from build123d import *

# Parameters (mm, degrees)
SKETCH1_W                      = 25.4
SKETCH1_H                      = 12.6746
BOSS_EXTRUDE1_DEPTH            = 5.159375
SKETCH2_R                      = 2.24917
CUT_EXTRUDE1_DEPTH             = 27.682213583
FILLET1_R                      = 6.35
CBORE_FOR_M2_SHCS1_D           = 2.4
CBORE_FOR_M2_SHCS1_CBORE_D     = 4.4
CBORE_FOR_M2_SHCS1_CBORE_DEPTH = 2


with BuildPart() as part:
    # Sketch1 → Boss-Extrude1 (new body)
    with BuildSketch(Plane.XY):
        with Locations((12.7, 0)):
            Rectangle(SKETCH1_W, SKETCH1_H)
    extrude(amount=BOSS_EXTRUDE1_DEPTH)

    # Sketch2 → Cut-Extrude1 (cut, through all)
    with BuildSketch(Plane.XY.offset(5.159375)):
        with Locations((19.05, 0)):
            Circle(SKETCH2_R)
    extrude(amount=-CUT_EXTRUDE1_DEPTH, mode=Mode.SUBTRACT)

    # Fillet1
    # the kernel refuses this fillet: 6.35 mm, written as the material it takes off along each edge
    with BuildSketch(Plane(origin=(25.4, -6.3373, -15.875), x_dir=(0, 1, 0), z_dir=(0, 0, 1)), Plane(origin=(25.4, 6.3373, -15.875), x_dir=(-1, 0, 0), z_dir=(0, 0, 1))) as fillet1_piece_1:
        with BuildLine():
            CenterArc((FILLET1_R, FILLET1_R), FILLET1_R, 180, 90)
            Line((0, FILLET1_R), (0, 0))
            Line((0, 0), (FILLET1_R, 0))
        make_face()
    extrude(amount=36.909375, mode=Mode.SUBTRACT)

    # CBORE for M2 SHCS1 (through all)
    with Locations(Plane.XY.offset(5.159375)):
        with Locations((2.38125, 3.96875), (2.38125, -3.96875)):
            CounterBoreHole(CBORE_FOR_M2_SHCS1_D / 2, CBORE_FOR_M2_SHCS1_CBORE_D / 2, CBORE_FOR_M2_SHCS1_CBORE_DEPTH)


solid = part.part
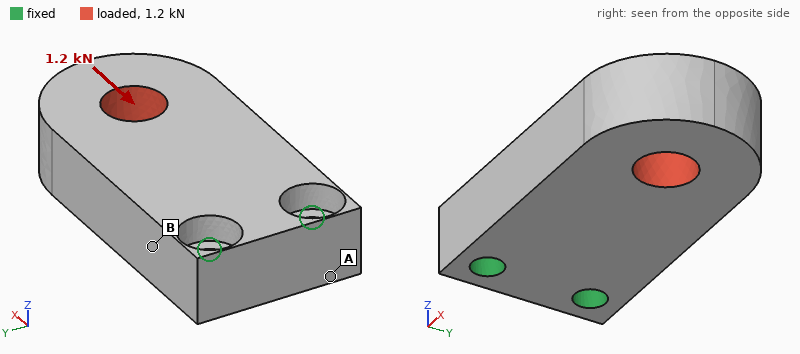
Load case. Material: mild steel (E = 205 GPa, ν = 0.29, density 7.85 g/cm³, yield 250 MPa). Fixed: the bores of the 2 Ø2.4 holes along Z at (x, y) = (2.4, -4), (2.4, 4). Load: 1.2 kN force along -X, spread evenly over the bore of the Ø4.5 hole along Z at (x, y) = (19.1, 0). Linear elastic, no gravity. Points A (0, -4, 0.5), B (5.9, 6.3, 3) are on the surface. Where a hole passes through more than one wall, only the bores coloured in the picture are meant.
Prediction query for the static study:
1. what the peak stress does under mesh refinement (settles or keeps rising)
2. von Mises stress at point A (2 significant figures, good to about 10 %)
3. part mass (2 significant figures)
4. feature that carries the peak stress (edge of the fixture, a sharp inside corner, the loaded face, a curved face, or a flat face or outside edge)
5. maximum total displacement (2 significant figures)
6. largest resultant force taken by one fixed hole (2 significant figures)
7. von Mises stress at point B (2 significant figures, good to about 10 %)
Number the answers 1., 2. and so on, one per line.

1. keeps rising
2. 10 MPa
3. 11 g
4. edge of the fixture
5. 7.1 µm
6. 600 N
7. 29 MPa
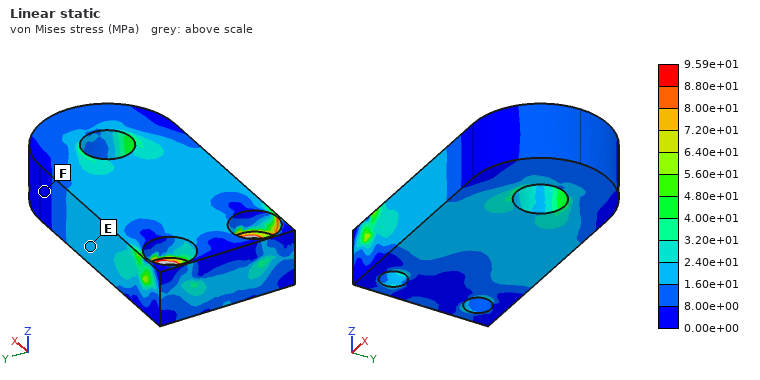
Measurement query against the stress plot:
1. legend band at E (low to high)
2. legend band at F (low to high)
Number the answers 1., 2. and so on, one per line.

1. 1.60e+01 to 2.40e+01 MPa
2. 0.00e+00 to 8.00e+00 MPa
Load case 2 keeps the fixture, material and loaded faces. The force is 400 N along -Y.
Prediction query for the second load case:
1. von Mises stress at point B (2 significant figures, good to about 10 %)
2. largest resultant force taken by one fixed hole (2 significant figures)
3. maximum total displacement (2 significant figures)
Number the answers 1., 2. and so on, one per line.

1. 41 MPa
2. 740 N
3. 8.7 µm
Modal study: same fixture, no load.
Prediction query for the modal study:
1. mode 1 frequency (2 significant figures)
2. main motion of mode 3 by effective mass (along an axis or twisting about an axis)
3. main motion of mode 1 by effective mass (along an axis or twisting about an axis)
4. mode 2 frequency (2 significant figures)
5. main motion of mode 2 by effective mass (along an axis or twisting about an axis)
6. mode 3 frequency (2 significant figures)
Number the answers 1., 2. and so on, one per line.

1. 6900 Hz
2. twisting about X
3. along Z
4. 17 kHz
5. along Y
6. 26 kHz
